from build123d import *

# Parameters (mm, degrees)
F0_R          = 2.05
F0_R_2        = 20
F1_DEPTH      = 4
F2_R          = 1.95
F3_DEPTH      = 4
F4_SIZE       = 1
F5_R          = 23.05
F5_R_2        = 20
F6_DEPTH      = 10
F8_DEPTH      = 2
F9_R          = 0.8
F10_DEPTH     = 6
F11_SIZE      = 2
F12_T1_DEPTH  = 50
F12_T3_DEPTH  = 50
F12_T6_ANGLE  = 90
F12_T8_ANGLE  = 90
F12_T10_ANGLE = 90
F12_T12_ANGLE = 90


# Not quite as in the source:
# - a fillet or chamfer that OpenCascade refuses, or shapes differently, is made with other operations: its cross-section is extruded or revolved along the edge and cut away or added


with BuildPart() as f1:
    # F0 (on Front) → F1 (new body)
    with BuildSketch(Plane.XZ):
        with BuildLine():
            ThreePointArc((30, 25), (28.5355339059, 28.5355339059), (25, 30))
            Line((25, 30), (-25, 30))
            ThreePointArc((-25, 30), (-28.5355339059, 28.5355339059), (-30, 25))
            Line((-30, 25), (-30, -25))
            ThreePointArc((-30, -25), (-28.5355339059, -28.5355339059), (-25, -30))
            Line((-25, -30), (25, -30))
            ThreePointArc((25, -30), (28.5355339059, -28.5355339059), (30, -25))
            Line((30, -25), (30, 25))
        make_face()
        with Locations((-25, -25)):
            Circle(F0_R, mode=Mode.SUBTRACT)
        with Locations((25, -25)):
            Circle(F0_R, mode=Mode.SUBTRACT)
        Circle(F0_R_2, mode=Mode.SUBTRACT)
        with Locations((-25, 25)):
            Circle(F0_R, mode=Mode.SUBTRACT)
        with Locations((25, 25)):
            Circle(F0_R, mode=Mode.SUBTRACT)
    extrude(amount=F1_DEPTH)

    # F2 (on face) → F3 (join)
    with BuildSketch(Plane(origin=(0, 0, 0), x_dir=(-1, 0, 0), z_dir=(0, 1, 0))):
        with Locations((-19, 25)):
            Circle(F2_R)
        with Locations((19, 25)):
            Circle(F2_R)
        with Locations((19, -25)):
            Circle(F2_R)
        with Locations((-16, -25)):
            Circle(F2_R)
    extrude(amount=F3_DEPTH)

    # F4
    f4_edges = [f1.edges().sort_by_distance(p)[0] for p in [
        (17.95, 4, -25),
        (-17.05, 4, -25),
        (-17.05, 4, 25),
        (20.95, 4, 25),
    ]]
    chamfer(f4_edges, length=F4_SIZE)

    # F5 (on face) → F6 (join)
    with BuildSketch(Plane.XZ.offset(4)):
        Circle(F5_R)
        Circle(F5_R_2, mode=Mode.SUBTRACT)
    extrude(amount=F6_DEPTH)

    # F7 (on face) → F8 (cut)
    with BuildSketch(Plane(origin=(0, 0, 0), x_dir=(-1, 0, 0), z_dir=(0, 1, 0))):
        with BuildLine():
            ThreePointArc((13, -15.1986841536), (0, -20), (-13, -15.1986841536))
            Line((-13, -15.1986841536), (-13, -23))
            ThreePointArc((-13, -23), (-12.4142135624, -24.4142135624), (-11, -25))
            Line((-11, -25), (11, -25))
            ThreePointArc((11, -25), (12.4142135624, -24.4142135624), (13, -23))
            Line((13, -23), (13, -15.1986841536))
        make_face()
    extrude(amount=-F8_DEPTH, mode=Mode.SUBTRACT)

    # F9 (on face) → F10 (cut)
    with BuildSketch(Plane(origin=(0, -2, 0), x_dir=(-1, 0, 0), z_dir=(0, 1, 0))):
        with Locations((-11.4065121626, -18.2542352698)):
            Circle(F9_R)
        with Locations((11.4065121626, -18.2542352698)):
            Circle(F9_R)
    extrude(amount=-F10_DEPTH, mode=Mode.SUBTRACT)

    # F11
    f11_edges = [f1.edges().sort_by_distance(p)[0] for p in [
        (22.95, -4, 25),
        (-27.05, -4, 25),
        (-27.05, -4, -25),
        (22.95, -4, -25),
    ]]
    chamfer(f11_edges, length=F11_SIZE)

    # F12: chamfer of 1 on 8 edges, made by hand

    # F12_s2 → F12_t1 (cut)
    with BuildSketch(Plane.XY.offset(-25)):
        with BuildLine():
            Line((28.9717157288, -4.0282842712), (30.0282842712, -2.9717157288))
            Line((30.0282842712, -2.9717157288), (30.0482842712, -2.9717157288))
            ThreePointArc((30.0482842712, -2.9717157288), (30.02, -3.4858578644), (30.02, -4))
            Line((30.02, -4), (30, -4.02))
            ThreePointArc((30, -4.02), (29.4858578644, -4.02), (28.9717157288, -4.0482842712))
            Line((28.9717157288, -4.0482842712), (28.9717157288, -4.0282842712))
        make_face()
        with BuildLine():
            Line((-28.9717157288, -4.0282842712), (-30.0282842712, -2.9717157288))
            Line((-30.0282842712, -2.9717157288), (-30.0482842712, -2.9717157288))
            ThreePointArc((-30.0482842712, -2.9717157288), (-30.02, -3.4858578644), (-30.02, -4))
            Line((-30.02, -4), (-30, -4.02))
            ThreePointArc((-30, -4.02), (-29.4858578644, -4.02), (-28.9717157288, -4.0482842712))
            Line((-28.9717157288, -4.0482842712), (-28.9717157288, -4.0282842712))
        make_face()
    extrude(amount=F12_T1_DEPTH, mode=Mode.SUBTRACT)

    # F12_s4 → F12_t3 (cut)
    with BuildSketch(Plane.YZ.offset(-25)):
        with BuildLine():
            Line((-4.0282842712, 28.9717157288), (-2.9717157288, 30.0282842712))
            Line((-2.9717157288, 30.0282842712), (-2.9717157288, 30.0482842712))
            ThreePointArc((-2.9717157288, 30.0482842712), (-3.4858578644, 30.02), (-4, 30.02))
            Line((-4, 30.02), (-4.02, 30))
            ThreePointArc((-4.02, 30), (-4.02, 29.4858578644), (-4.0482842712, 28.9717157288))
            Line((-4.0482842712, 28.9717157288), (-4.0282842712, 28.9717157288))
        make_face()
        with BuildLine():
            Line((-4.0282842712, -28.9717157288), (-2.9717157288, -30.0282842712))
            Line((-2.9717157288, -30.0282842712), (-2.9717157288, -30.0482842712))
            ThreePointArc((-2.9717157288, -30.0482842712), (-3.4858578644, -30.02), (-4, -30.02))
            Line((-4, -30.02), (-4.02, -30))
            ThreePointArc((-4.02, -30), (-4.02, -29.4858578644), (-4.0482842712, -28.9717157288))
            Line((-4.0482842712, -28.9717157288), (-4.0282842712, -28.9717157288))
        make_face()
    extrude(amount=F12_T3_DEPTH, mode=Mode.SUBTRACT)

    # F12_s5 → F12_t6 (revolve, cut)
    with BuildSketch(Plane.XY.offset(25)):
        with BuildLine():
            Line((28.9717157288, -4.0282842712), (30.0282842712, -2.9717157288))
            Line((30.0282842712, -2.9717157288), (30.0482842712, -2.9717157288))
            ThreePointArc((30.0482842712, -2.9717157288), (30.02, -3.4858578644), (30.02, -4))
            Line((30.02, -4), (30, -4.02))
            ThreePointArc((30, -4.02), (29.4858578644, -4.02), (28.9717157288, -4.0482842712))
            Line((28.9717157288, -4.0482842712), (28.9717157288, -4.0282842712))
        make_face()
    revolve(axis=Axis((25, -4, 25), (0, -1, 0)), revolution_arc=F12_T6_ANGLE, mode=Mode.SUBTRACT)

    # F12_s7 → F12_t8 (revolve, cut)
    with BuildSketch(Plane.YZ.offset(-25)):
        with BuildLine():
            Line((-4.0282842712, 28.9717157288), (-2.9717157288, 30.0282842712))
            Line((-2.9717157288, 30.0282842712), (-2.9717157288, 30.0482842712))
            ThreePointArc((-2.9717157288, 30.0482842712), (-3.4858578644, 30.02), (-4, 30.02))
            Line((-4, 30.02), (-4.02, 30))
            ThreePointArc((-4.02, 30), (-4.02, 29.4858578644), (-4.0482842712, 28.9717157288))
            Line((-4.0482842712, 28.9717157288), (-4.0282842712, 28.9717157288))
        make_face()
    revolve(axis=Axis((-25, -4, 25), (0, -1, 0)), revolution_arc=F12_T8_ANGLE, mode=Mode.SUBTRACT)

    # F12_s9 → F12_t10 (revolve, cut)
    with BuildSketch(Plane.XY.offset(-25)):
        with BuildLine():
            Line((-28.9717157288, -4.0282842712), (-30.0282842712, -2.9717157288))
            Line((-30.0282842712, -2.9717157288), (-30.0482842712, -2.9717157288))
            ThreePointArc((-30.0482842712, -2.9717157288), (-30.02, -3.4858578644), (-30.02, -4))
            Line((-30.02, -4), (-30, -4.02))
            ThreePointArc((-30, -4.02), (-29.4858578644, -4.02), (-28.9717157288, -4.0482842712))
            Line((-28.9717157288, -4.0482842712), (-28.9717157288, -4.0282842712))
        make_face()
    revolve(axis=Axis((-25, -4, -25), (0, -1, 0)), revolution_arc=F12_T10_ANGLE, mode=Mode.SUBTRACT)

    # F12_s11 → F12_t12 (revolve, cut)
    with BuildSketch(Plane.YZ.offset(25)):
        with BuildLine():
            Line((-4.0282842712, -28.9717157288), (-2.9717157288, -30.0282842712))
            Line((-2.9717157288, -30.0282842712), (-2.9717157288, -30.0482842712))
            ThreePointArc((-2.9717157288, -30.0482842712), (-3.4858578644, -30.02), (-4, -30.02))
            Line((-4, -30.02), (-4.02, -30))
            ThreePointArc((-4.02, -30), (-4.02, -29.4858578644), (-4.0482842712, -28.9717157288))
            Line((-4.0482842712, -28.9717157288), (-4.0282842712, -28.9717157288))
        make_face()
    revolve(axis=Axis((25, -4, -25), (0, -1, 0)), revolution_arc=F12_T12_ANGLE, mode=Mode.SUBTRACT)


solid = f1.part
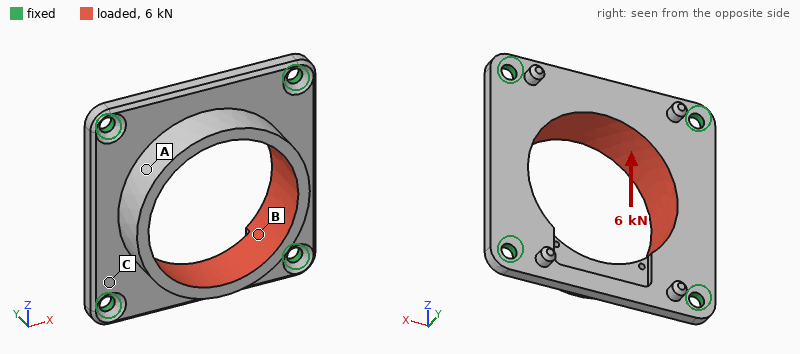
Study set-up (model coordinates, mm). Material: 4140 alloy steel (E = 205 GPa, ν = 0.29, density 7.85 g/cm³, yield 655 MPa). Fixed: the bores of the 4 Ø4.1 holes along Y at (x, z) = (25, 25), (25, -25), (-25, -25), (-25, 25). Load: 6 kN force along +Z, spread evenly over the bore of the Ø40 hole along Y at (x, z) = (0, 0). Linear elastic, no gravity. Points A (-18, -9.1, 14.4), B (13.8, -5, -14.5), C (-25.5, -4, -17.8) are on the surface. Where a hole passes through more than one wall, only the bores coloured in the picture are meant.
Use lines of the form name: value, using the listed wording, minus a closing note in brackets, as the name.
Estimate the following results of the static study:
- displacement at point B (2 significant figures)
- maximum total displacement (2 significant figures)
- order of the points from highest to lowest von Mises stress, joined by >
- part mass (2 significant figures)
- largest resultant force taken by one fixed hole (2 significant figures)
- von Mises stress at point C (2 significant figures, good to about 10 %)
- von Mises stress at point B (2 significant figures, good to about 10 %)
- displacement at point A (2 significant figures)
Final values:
displacement at point B: 6.7 µm
maximum total displacement: 19 µm
order of the points from highest to lowest von Mises stress, joined by >: B > C > A
part mass: 100 g
largest resultant force taken by one fixed hole: 1.6 kN
von Mises stress at point C: 31 MPa
von Mises stress at point B: 43 MPa
displacement at point A: 7.3 µm
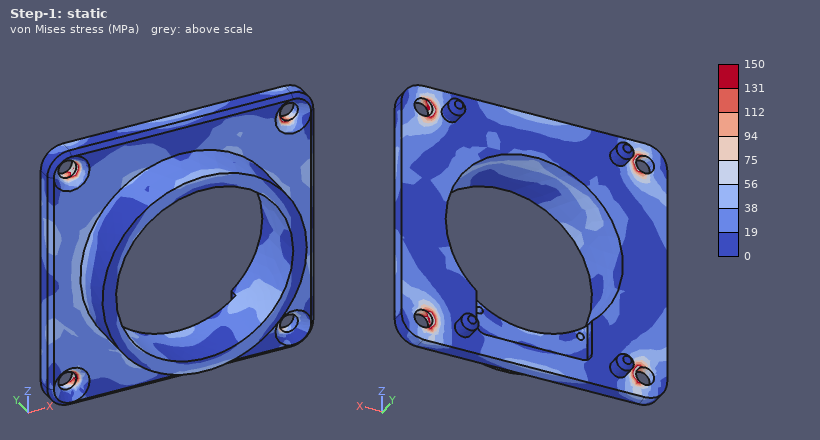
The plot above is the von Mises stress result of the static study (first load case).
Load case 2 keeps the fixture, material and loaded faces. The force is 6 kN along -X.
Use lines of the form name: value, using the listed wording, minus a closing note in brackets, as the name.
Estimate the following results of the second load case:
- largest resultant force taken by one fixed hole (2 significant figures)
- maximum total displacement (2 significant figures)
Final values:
largest resultant force taken by one fixed hole: 1.7 kN
maximum total displacement: 18 µm
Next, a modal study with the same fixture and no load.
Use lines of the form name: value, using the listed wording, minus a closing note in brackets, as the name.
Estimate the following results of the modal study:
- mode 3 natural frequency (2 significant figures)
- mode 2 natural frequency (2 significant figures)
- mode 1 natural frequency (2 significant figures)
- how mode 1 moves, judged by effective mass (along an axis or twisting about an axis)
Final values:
mode 3 natural frequency: 8500 Hz
mode 2 natural frequency: 8400 Hz
mode 1 natural frequency: 7200 Hz
how mode 1 moves, judged by effective mass: along Y
